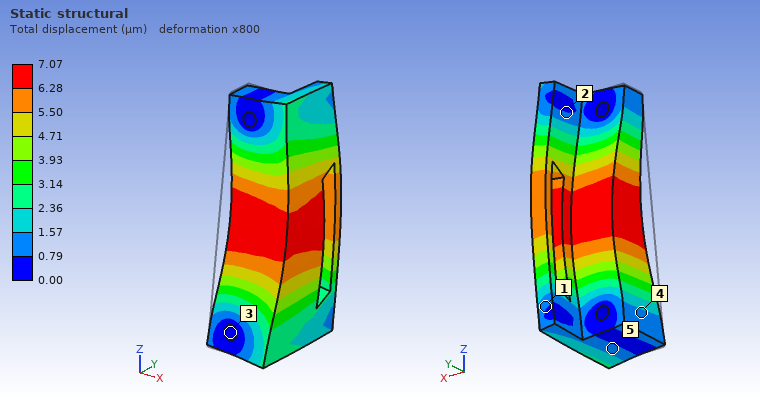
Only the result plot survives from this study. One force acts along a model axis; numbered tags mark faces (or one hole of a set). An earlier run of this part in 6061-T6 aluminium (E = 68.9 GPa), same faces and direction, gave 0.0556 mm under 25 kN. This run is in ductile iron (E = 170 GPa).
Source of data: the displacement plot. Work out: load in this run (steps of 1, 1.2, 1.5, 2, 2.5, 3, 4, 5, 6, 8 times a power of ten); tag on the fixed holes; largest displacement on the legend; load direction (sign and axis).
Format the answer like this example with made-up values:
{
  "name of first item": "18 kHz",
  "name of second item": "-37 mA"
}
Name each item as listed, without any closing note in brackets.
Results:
{
  "load in this run": "8 kN",
  "tag on the fixed holes": "3",
  "largest displacement on the legend": "7.07 µm",
  "load direction": "+X"
}
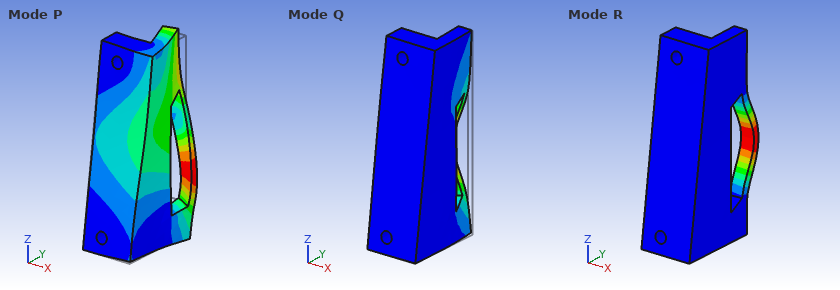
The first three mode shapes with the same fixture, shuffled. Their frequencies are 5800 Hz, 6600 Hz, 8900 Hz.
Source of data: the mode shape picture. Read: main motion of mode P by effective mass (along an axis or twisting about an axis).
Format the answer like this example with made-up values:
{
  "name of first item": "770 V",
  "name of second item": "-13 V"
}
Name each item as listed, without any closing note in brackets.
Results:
{
  "main motion of mode P by effective mass": "along Y"
}
